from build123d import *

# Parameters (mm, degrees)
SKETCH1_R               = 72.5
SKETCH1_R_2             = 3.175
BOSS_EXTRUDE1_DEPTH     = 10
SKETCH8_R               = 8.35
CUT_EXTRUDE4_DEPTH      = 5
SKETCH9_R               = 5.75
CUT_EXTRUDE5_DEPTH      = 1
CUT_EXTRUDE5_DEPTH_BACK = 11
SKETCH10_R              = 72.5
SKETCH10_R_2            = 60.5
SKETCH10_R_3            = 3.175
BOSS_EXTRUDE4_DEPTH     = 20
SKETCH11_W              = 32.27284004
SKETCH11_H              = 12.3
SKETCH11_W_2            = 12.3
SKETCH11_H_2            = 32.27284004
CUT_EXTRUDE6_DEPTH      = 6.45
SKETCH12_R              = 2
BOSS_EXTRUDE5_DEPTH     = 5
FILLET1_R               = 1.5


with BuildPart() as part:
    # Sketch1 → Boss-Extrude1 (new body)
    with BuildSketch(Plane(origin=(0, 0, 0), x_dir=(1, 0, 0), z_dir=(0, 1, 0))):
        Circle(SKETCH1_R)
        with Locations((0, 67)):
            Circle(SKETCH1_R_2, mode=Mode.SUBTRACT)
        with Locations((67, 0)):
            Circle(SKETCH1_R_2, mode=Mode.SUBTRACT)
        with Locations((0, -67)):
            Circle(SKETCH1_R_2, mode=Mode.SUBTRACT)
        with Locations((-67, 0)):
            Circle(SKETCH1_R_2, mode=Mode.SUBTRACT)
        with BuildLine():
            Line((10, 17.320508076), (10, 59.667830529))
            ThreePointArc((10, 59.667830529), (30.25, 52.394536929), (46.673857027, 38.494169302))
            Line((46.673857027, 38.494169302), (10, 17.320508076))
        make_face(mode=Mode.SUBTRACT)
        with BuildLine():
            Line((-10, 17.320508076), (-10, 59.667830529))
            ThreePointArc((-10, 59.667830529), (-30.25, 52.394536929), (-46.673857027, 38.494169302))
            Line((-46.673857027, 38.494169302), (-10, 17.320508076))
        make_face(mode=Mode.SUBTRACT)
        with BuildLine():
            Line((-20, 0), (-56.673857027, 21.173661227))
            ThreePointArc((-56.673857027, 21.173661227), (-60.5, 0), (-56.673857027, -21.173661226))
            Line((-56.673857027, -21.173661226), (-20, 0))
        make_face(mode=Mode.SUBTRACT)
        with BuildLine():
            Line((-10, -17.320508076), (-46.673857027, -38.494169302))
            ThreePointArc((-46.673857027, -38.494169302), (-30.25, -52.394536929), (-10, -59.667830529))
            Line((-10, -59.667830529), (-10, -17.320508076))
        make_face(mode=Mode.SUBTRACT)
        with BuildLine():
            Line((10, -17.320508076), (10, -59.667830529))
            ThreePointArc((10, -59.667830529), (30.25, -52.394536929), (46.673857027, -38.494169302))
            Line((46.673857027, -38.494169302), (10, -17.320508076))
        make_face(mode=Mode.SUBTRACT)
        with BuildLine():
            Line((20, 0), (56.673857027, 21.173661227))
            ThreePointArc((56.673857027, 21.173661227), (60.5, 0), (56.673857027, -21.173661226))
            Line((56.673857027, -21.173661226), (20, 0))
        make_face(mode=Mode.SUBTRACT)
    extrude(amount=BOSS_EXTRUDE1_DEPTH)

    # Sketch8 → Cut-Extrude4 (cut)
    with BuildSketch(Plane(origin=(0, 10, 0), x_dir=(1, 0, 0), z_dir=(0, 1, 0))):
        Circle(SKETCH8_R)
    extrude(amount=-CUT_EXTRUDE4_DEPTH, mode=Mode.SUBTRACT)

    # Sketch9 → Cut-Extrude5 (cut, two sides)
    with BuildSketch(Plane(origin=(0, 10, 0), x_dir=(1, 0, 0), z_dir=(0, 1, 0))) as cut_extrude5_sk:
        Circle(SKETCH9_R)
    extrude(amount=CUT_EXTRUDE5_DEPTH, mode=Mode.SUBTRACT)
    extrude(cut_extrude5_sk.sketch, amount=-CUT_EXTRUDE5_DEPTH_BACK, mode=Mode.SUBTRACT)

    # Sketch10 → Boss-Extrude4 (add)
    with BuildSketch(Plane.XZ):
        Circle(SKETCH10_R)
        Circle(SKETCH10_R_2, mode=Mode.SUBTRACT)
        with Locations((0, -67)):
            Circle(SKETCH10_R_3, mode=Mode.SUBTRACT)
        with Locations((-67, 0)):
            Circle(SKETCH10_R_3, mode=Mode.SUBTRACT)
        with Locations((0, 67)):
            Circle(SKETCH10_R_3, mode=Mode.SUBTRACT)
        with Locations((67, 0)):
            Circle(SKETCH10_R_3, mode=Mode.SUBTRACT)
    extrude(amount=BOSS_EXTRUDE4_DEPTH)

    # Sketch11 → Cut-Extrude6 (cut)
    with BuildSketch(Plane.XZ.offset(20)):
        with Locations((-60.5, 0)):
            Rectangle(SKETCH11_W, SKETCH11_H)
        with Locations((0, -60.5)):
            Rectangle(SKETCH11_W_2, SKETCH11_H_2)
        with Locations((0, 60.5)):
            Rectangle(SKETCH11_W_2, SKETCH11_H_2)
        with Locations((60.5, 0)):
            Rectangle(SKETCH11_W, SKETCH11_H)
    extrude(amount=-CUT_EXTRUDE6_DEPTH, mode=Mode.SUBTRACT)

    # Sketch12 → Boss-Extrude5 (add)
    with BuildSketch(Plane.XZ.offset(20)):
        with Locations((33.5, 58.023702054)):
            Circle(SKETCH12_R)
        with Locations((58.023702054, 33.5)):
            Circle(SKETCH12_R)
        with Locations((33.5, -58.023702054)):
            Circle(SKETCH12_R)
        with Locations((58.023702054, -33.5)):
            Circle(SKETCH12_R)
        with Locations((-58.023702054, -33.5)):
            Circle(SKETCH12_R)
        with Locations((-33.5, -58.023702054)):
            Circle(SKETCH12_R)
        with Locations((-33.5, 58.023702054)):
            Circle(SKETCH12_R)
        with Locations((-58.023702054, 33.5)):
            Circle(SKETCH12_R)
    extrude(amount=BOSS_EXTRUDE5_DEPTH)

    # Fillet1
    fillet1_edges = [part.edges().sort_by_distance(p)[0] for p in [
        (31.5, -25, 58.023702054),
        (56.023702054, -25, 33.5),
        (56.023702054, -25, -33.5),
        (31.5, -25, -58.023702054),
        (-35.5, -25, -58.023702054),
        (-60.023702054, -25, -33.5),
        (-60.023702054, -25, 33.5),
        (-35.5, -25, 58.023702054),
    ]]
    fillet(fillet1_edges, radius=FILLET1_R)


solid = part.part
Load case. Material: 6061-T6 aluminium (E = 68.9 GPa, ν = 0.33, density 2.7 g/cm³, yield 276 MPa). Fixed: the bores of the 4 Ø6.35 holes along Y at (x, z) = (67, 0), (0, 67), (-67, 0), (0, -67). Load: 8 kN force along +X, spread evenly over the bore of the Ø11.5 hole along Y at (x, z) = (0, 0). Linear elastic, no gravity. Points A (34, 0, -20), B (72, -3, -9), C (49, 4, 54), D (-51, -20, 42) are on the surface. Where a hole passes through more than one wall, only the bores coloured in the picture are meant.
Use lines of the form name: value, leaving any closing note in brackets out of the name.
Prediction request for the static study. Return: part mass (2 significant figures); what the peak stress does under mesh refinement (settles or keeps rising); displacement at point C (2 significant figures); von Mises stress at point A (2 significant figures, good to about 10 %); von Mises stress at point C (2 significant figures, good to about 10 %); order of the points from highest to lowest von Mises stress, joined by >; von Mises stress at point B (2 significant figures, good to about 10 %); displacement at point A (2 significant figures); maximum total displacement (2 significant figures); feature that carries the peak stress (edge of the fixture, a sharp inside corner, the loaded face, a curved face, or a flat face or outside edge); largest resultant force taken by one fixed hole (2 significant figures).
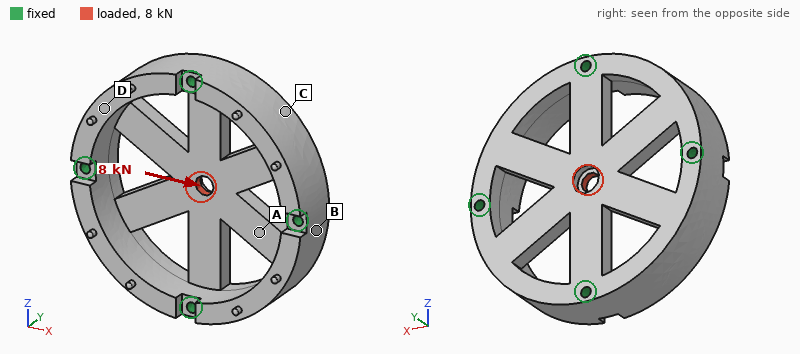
part mass: 550 g
what the peak stress does under mesh refinement: keeps rising
displacement at point C: 8.6 µm
von Mises stress at point A: 19 MPa
von Mises stress at point C: 7.2 MPa
order of the points from highest to lowest von Mises stress, joined by >: A > B > C > D
von Mises stress at point B: 11 MPa
displacement at point A: 20 µm
maximum total displacement: 32 µm
feature that carries the peak stress: a sharp inside corner
largest resultant force taken by one fixed hole: 2.8 kN
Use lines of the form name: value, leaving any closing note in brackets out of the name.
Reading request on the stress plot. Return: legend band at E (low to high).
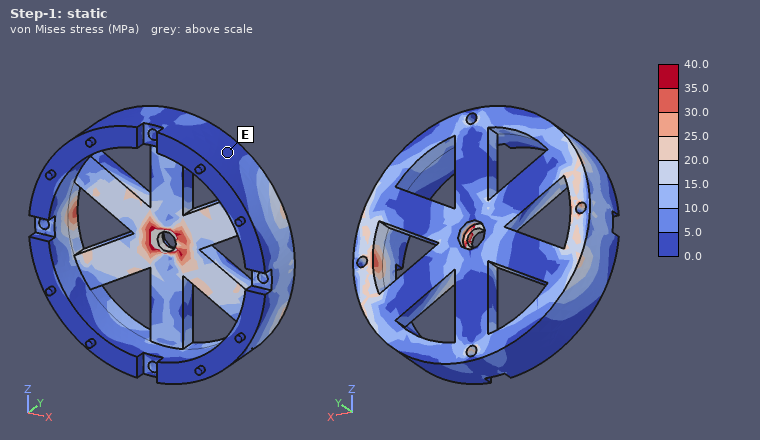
legend band at E: 0.0 to 5.0 MPa
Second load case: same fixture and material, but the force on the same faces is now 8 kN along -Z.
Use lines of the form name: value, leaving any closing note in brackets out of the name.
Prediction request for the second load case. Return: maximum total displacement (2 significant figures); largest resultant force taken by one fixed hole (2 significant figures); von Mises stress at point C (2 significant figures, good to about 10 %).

maximum total displacement: 20 µm
largest resultant force taken by one fixed hole: 2.8 kN
von Mises stress at point C: 4.2 MPa
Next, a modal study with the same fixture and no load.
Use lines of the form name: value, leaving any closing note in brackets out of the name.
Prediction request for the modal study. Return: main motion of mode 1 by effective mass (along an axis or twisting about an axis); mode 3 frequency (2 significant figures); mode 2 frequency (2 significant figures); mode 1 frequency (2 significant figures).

main motion of mode 1 by effective mass: along Y
mode 3 frequency: 7400 Hz
mode 2 frequency: 7100 Hz
mode 1 frequency: 3700 Hz
